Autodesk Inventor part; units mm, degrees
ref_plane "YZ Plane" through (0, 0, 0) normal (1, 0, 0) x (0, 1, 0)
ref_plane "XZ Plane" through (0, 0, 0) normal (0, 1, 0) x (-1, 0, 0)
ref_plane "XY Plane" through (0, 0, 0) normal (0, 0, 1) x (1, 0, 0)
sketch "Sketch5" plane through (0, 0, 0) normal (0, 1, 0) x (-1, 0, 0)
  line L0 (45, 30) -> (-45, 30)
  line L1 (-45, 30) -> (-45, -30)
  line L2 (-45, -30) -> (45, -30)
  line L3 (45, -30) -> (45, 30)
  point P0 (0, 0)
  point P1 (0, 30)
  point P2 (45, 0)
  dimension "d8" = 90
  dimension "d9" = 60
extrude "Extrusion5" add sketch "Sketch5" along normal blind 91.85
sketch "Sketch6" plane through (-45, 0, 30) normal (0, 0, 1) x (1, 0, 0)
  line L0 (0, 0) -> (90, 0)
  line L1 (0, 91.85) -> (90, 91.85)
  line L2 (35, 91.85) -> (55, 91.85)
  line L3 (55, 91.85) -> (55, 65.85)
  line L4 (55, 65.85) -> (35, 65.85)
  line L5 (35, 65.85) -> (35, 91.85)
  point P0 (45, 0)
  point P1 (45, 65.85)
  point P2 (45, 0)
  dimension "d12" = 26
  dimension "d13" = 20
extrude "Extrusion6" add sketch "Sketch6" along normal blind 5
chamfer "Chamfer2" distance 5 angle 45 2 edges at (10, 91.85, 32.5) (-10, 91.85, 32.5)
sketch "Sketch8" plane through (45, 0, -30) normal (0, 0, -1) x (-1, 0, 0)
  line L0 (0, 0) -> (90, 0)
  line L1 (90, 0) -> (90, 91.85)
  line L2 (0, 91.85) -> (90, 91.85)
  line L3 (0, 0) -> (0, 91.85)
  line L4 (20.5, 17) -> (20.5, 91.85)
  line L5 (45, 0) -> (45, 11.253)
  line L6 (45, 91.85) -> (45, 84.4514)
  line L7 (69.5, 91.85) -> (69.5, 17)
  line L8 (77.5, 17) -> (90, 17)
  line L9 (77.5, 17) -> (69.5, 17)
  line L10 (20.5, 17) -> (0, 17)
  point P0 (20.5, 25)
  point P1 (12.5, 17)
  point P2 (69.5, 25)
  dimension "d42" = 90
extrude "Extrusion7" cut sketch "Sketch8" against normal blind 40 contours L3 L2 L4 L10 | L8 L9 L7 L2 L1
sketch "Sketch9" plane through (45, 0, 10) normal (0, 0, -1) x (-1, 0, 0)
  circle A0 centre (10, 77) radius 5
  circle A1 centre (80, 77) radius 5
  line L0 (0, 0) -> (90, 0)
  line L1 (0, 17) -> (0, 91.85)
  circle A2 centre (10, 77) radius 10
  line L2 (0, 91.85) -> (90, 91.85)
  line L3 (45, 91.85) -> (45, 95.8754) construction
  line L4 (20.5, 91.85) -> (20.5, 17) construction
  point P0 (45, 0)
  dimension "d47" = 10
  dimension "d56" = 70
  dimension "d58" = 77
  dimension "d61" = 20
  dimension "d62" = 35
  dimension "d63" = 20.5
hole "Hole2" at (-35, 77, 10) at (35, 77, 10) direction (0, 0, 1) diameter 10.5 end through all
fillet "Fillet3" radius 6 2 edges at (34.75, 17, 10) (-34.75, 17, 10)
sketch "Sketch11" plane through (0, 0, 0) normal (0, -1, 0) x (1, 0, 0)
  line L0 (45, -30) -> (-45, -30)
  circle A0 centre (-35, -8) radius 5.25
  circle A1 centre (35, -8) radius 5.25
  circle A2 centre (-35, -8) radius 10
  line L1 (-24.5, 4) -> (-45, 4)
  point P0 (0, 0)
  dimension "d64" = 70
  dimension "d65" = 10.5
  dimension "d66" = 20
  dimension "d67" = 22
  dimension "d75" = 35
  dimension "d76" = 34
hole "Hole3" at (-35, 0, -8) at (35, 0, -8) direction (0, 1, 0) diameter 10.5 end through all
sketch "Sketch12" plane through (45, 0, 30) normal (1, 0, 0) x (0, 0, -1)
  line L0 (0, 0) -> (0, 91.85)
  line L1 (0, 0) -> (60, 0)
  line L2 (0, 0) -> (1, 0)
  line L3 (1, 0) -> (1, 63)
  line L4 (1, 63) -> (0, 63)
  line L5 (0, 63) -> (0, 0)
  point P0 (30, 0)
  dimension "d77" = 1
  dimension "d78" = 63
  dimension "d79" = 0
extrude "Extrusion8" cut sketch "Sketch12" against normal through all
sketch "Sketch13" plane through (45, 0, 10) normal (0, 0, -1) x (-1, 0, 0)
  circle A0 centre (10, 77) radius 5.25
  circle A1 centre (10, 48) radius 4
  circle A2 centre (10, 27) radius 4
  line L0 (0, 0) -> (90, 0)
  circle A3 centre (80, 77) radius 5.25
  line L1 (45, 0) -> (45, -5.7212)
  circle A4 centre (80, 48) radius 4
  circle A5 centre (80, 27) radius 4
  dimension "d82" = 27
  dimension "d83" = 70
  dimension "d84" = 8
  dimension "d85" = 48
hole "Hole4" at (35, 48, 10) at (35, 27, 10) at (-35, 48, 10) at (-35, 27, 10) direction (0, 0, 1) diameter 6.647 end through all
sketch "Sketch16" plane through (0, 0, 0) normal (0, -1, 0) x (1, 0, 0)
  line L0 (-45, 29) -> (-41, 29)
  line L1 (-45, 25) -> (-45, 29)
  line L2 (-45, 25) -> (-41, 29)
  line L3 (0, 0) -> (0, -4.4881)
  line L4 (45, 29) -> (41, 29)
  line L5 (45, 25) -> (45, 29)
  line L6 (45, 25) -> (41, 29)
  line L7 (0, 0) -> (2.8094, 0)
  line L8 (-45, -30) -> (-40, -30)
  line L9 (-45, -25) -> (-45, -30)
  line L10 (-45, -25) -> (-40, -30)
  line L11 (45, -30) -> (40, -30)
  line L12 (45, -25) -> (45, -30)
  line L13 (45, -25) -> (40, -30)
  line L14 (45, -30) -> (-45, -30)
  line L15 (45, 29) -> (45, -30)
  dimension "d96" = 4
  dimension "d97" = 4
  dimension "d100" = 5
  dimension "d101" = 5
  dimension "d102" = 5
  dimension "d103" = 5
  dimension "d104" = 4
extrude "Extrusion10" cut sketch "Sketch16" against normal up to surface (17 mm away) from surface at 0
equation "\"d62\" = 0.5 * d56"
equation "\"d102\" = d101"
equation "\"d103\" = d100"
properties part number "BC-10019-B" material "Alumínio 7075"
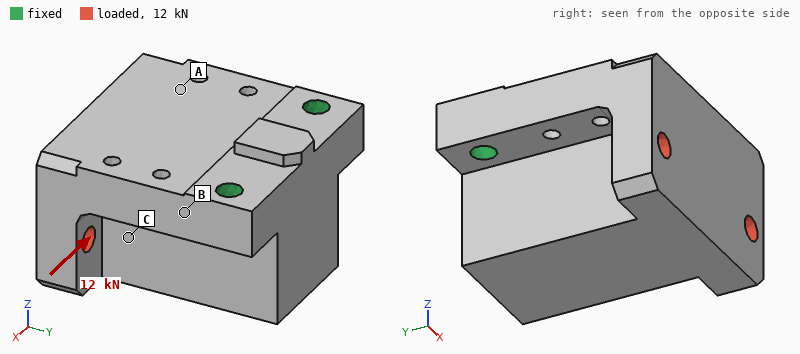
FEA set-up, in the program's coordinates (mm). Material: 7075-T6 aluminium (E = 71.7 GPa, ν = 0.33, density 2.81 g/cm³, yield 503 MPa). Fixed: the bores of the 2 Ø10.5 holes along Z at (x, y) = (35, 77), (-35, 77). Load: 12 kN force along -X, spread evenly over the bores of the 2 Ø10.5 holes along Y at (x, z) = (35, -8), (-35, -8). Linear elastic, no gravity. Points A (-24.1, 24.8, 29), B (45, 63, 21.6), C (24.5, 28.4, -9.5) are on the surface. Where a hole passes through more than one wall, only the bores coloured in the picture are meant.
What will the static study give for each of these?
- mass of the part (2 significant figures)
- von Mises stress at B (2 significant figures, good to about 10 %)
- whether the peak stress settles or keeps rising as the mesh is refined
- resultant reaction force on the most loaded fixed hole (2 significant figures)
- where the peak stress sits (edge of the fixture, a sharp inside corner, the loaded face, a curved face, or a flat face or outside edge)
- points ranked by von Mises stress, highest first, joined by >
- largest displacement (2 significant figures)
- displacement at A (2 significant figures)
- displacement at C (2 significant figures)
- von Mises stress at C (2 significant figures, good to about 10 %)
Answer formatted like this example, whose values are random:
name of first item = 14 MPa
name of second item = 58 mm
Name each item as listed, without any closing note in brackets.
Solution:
mass of the part = 1.0 kg
von Mises stress at B = 22 MPa
whether the peak stress settles or keeps rising as the mesh is refined = keeps rising
resultant reaction force on the most loaded fixed hole = 14 kN
where the peak stress sits = edge of the fixture
points ranked by von Mises stress, highest first, joined by > = B > C > A
largest displacement = 58 µm
displacement at A = 18 µm
displacement at C = 32 µm
von Mises stress at C = 9.0 MPa
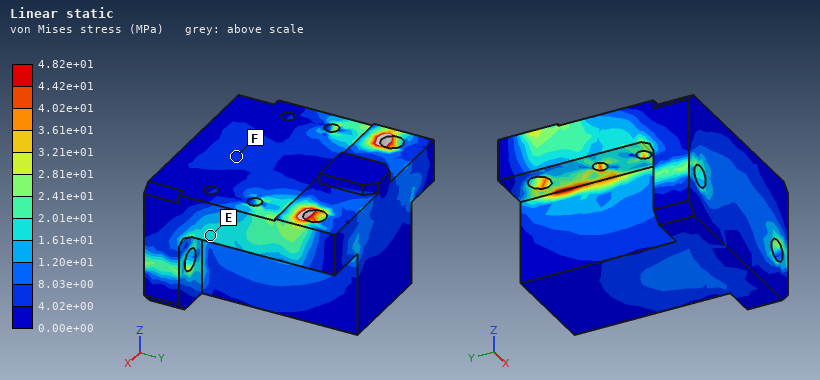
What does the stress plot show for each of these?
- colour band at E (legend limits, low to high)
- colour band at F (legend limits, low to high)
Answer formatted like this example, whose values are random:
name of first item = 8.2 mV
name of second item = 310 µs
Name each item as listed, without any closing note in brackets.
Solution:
colour band at E = 1.61e+01 to 2.01e+01 MPa
colour band at F = 4.02e+00 to 8.03e+00 MPa
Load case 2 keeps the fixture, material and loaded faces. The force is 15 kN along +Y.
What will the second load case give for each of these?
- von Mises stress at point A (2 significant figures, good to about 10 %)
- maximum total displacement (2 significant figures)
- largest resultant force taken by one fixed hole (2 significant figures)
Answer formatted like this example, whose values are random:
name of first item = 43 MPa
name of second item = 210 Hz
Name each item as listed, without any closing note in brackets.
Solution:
von Mises stress at point A = 9.6 MPa
maximum total displacement = 0.17 mm
largest resultant force taken by one fixed hole = 7.7 kN
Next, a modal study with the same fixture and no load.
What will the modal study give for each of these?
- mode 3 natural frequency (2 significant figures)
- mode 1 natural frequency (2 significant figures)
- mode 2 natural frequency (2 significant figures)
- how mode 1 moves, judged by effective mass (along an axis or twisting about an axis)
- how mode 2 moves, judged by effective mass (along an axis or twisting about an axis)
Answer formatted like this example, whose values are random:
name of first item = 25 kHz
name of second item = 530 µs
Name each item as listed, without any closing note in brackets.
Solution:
mode 3 natural frequency = 6000 Hz
mode 1 natural frequency = 1600 Hz
mode 2 natural frequency = 4300 Hz
how mode 1 moves, judged by effective mass = along Z
how mode 2 moves, judged by effective mass = along X
